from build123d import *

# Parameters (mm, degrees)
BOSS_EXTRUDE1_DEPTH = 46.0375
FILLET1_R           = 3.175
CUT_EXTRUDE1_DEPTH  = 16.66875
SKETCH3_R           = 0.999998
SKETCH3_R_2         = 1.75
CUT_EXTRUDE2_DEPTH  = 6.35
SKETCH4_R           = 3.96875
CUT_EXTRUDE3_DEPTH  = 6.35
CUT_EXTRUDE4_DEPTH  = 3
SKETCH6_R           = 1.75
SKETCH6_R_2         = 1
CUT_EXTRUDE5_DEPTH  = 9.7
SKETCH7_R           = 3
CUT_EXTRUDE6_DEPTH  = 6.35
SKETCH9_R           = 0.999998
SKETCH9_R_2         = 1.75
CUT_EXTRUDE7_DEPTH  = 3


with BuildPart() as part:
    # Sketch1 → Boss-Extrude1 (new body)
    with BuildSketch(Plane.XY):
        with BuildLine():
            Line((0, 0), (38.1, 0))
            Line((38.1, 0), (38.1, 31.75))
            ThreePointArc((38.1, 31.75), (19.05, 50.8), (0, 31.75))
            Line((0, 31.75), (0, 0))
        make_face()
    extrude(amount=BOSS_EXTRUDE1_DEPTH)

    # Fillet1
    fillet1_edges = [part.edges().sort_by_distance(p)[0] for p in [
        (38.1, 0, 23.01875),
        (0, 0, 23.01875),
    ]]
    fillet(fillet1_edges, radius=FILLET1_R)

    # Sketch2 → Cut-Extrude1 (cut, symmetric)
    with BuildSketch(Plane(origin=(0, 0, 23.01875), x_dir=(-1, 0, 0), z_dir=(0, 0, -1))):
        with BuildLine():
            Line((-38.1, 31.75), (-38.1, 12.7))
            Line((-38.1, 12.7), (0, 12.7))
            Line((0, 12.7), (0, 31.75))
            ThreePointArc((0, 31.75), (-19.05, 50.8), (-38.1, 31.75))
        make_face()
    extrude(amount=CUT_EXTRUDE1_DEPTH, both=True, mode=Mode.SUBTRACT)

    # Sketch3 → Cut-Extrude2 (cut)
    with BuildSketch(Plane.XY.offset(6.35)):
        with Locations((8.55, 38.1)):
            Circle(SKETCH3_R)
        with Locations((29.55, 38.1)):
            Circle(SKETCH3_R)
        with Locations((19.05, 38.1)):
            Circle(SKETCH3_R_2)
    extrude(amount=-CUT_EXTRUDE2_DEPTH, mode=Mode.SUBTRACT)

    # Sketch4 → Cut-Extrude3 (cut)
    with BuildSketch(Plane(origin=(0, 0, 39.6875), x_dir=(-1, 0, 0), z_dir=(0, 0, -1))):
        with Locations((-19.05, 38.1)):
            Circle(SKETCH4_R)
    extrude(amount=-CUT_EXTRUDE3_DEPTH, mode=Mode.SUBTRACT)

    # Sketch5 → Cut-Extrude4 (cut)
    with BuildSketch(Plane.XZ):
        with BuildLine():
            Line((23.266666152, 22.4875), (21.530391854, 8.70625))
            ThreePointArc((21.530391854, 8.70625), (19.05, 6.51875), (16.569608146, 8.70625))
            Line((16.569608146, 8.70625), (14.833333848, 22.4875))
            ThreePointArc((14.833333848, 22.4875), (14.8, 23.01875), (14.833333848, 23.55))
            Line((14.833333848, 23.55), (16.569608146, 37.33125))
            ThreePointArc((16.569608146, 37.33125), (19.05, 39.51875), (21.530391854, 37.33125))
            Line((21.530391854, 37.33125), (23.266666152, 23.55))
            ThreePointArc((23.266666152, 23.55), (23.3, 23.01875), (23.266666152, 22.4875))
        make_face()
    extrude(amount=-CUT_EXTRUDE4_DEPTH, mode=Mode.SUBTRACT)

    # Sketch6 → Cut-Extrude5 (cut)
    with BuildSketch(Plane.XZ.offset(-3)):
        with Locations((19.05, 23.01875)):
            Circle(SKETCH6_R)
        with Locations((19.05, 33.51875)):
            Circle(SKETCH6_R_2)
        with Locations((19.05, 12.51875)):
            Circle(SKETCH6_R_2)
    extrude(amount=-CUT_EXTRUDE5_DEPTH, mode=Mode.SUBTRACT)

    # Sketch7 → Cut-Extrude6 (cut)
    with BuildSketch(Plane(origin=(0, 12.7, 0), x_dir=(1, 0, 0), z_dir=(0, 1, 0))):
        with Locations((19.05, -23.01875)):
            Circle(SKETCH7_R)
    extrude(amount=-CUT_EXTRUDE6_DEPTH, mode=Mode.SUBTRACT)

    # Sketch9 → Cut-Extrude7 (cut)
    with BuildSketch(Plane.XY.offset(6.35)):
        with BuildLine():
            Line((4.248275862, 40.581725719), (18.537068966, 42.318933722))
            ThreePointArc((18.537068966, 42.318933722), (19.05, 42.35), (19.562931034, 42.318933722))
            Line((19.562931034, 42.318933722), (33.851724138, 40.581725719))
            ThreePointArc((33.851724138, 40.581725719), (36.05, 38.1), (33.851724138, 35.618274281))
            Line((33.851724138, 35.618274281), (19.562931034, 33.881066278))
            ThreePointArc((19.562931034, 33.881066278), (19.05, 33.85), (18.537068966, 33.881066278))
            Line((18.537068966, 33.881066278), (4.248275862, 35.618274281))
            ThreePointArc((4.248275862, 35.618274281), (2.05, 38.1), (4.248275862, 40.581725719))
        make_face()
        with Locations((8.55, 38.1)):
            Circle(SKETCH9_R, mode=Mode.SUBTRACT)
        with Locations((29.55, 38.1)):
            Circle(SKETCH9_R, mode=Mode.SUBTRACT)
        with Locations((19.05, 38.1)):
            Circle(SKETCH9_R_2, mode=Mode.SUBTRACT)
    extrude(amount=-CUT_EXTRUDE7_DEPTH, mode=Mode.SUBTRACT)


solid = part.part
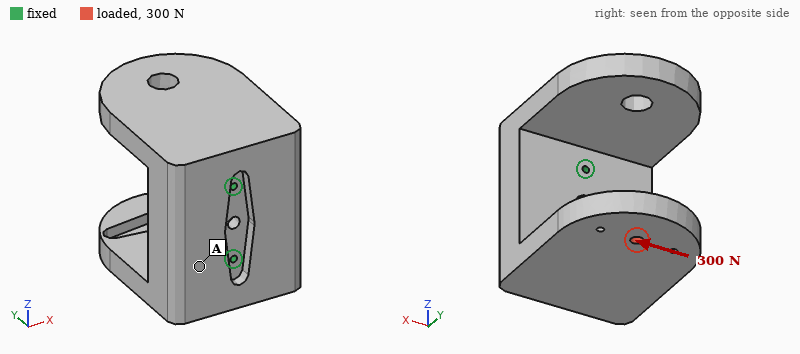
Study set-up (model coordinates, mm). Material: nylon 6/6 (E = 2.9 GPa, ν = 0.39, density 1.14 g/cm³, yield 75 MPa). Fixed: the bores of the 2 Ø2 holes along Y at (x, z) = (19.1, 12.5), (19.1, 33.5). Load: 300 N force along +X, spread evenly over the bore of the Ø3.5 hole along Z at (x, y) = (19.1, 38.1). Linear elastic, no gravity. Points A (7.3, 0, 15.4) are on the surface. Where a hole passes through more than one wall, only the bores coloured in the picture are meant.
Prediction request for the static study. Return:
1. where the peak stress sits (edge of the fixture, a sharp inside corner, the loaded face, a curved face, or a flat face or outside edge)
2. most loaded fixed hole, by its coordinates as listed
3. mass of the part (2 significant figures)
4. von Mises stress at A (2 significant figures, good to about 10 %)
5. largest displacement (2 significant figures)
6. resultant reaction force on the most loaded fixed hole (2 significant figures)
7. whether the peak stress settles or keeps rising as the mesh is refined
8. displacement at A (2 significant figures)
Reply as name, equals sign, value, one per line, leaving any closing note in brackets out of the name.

where the peak stress sits = edge of the fixture
most loaded fixed hole, by its coordinates as listed = (19.1, 12.5)
mass of the part = 42 g
von Mises stress at A = 4.8 MPa
largest displacement = 0.64 mm
resultant reaction force on the most loaded fixed hole = 450 N
whether the peak stress settles or keeps rising as the mesh is refined = keeps rising
displacement at A = 0.13 mm
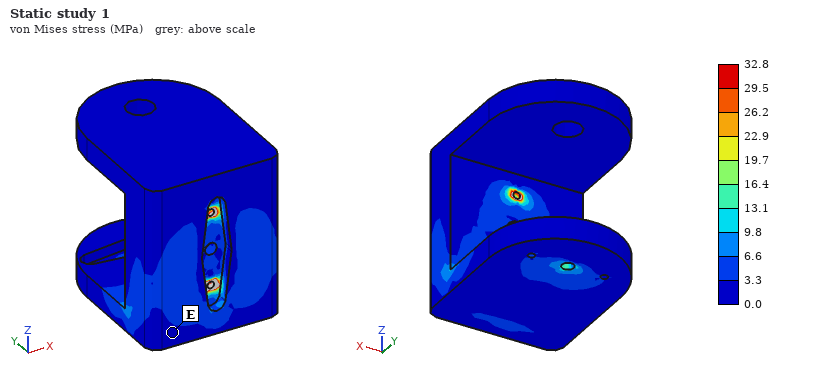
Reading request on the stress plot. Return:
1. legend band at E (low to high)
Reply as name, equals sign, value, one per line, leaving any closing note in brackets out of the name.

legend band at E = 0.0 to 3.3 MPa
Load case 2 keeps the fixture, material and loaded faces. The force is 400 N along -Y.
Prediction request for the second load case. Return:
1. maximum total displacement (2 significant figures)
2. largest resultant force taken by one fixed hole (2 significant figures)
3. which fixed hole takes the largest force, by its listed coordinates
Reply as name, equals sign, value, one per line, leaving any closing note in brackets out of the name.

maximum total displacement = 0.38 mm
largest resultant force taken by one fixed hole = 510 N
which fixed hole takes the largest force, by its listed coordinates = (19.1, 12.5)
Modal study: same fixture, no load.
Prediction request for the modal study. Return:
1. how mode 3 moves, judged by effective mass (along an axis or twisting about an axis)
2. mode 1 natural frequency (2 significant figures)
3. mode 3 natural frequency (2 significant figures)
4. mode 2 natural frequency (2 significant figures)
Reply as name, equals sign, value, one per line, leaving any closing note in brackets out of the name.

how mode 3 moves, judged by effective mass = along X
mode 1 natural frequency = 1100 Hz
mode 3 natural frequency = 1300 Hz
mode 2 natural frequency = 1100 Hz
